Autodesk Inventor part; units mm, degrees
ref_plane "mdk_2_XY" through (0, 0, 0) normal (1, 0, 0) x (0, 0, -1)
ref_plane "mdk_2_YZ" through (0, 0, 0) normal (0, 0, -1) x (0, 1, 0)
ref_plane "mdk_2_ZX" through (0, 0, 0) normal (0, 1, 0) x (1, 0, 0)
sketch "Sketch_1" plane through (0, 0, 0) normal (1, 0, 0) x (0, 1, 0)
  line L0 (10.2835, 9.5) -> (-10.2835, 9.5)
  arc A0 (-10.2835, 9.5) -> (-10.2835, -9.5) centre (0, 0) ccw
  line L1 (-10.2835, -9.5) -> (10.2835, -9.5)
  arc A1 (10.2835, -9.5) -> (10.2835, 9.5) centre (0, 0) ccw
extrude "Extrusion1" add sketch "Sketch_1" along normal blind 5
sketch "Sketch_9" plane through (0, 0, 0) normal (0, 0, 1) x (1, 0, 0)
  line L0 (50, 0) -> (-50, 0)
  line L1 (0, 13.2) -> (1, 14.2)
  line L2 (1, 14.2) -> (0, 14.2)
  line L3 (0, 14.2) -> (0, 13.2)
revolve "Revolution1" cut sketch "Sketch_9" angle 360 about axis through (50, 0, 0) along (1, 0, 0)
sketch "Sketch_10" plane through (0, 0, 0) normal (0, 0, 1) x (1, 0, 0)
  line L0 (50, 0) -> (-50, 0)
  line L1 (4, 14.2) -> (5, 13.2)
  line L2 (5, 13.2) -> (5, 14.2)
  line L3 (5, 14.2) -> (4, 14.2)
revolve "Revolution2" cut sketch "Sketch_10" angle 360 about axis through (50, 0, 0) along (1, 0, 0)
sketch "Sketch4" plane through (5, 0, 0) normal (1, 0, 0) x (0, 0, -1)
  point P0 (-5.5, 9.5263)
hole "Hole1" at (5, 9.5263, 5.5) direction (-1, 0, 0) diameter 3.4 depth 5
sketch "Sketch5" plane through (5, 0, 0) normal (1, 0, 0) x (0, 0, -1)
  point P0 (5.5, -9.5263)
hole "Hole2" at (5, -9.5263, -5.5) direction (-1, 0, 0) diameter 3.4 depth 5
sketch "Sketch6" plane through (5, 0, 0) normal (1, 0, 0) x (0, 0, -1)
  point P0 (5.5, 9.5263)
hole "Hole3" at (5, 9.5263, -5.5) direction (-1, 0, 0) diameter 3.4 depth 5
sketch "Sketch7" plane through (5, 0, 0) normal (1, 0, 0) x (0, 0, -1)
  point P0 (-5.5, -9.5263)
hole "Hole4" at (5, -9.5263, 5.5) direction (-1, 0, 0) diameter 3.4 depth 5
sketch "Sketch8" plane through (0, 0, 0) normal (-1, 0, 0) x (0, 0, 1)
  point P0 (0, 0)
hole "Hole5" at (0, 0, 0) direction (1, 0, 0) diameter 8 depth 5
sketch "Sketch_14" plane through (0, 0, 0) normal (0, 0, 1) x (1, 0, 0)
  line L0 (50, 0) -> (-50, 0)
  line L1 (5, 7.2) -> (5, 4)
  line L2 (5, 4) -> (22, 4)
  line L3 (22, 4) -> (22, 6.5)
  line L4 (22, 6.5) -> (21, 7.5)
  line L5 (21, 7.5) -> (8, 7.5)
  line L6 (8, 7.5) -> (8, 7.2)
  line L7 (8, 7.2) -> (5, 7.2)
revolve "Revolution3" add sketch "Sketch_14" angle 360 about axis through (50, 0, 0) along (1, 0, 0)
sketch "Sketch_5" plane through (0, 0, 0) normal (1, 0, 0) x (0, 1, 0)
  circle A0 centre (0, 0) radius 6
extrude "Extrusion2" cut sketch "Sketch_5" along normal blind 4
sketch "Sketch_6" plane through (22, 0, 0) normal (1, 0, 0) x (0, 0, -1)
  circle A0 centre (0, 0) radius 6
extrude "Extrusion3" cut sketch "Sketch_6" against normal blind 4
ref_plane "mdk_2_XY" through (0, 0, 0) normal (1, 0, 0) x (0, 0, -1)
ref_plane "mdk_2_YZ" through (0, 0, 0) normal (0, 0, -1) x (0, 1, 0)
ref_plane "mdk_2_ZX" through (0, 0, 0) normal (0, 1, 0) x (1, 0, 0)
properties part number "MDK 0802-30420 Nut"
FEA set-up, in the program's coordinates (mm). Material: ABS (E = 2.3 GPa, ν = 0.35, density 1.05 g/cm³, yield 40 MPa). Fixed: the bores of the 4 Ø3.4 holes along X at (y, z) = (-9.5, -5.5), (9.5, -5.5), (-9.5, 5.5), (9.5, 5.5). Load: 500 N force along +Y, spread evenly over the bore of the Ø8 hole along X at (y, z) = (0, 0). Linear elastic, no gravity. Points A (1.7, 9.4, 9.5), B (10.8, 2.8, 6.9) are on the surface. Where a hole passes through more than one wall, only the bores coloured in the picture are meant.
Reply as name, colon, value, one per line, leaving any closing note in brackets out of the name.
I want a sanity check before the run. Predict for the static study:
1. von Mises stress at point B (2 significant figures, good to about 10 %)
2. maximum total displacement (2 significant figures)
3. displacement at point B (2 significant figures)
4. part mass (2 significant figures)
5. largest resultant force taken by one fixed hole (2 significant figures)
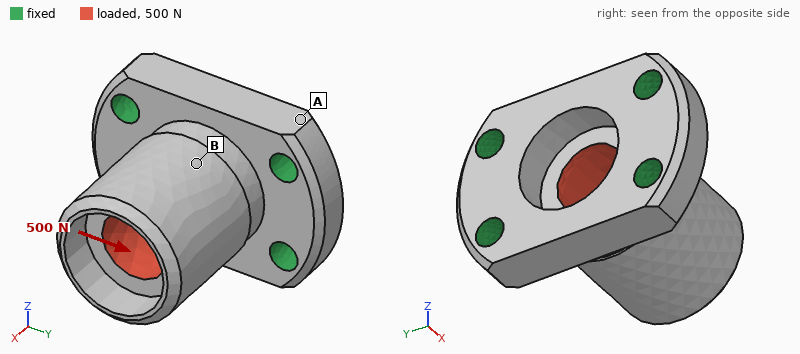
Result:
von Mises stress at point B: 4.5 MPa
maximum total displacement: 0.16 mm
displacement at point B: 0.071 mm
part mass: 3.7 g
largest resultant force taken by one fixed hole: 190 N
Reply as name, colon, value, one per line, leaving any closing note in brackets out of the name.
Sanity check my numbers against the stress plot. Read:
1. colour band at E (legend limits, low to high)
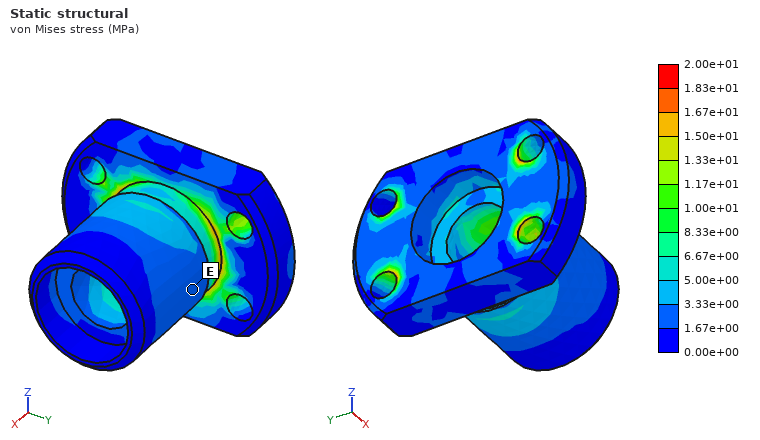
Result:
colour band at E: 1.67e+00 to 3.33e+00 MPa
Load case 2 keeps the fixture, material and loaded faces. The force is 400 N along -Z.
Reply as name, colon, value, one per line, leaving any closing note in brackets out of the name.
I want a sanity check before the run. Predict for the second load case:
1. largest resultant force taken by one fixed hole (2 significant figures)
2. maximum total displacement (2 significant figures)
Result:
largest resultant force taken by one fixed hole: 180 N
maximum total displacement: 0.20 mm
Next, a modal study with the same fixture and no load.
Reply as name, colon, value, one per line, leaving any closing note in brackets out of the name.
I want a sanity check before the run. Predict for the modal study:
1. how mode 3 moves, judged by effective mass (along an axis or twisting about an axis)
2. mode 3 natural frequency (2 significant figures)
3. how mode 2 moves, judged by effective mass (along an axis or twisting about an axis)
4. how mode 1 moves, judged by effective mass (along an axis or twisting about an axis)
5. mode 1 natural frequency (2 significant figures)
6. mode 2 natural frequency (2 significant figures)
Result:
how mode 3 moves, judged by effective mass: twisting about X
mode 3 natural frequency: 12 kHz
how mode 2 moves, judged by effective mass: along Y
how mode 1 moves, judged by effective mass: along Z
mode 1 natural frequency: 5300 Hz
mode 2 natural frequency: 6600 Hz
